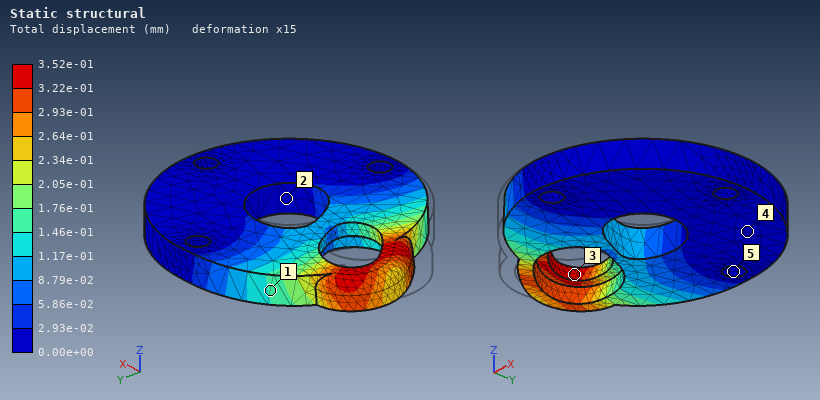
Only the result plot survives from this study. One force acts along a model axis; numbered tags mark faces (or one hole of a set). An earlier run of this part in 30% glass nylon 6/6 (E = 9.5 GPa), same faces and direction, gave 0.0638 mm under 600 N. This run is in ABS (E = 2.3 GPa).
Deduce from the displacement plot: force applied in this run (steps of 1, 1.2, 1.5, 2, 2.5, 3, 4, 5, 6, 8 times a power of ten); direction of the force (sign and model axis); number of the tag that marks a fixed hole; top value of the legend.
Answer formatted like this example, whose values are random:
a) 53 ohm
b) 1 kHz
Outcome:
a) 800 N
b) +Y
c) 5
d) 3.52e-01 mm
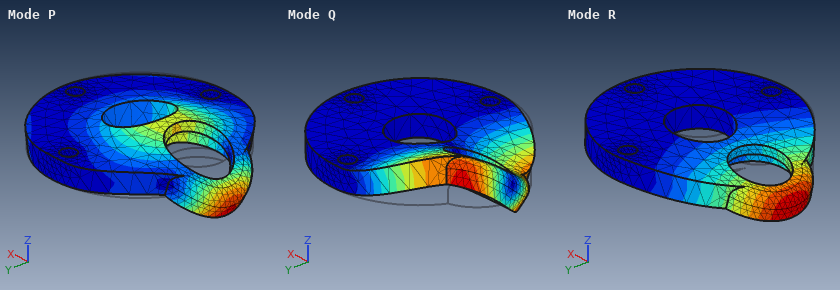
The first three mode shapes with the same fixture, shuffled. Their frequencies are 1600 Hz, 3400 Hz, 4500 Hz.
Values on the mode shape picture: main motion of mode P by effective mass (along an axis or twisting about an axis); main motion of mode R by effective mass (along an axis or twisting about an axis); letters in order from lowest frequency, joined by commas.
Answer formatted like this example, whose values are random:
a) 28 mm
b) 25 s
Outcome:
a) along Z
b) along Z
c) R, Q, P
